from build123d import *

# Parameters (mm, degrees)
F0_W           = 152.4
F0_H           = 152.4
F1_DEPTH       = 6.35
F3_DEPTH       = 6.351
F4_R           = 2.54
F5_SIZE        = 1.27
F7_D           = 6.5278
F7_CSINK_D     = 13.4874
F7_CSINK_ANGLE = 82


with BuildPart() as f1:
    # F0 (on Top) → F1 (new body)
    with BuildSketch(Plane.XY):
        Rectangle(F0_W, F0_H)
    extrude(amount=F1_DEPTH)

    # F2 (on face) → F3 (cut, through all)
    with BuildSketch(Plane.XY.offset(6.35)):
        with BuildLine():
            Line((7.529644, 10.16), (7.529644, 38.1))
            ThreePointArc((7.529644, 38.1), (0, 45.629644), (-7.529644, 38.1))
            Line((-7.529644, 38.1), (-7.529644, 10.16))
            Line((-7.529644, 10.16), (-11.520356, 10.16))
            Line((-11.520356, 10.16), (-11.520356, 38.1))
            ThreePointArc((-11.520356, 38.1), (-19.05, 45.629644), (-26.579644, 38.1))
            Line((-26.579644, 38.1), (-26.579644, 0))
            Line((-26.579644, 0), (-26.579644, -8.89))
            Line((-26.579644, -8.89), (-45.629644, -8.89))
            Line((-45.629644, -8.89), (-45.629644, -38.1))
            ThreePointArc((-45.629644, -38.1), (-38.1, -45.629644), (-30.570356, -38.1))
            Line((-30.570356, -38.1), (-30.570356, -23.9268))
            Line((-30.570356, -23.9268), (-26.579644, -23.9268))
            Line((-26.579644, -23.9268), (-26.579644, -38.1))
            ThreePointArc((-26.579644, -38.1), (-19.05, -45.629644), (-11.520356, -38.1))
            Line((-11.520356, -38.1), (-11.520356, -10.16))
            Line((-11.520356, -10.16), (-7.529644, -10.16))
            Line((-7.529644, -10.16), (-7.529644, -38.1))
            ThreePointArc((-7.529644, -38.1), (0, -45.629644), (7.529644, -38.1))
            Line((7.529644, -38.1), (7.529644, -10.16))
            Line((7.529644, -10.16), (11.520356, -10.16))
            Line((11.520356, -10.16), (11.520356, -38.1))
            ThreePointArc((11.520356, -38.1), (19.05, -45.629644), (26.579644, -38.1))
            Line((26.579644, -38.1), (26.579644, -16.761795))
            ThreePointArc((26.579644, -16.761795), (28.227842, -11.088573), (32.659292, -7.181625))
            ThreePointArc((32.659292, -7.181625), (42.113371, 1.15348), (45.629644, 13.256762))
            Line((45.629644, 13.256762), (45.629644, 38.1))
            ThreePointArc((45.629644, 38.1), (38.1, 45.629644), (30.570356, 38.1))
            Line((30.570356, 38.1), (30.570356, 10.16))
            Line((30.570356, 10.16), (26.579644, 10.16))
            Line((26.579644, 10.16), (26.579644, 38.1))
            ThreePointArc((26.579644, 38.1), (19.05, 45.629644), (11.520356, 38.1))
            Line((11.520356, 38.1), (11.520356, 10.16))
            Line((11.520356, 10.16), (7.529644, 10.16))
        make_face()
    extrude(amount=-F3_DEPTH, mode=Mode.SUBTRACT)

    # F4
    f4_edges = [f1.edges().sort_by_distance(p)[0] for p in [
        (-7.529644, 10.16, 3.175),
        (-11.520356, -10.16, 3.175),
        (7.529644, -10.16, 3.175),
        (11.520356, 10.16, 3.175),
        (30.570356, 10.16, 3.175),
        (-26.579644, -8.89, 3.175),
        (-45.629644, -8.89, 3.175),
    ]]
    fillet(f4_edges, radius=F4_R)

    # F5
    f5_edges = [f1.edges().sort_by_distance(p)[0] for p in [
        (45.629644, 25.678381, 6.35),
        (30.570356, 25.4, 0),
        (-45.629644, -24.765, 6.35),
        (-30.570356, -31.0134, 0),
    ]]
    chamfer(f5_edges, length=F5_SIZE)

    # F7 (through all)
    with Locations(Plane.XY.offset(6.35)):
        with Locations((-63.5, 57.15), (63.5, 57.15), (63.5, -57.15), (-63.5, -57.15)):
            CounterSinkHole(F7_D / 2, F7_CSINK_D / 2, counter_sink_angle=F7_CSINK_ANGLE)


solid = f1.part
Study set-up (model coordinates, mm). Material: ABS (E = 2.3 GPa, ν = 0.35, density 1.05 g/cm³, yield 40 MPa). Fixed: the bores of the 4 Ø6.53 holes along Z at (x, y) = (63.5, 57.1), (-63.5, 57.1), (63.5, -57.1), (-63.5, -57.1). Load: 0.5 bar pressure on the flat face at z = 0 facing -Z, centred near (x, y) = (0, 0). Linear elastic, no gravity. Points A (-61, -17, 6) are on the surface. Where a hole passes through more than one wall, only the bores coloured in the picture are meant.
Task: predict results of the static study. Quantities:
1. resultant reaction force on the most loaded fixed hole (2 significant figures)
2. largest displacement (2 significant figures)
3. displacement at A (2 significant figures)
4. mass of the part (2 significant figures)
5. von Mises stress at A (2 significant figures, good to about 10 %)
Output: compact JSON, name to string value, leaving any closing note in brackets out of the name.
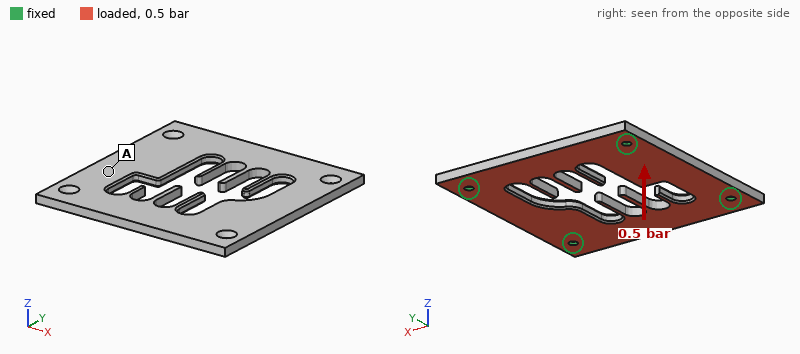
{"resultant reaction force on the most loaded fixed hole": "340 N", "largest displacement": "2.5 mm", "displacement at A": "0.73 mm", "mass of the part": "120 g", "von Mises stress at A": "5.6 MPa"}
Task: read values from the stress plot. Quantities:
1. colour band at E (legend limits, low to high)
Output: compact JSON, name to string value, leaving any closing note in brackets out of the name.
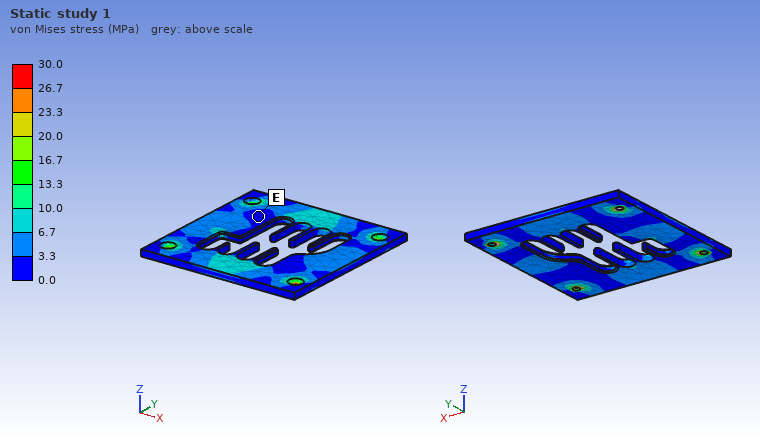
{"colour band at E": "0.0 to 3.3 MPa"}
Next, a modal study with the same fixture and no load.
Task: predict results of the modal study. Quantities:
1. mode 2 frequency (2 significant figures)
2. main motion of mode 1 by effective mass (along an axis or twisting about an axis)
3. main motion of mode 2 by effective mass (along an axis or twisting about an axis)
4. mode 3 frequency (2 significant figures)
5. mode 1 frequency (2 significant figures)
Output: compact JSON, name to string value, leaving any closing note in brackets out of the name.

{"mode 2 frequency": "470 Hz", "main motion of mode 1 by effective mass": "along Z", "main motion of mode 2 by effective mass": "twisting about X", "mode 3 frequency": "540 Hz", "mode 1 frequency": "400 Hz"}
